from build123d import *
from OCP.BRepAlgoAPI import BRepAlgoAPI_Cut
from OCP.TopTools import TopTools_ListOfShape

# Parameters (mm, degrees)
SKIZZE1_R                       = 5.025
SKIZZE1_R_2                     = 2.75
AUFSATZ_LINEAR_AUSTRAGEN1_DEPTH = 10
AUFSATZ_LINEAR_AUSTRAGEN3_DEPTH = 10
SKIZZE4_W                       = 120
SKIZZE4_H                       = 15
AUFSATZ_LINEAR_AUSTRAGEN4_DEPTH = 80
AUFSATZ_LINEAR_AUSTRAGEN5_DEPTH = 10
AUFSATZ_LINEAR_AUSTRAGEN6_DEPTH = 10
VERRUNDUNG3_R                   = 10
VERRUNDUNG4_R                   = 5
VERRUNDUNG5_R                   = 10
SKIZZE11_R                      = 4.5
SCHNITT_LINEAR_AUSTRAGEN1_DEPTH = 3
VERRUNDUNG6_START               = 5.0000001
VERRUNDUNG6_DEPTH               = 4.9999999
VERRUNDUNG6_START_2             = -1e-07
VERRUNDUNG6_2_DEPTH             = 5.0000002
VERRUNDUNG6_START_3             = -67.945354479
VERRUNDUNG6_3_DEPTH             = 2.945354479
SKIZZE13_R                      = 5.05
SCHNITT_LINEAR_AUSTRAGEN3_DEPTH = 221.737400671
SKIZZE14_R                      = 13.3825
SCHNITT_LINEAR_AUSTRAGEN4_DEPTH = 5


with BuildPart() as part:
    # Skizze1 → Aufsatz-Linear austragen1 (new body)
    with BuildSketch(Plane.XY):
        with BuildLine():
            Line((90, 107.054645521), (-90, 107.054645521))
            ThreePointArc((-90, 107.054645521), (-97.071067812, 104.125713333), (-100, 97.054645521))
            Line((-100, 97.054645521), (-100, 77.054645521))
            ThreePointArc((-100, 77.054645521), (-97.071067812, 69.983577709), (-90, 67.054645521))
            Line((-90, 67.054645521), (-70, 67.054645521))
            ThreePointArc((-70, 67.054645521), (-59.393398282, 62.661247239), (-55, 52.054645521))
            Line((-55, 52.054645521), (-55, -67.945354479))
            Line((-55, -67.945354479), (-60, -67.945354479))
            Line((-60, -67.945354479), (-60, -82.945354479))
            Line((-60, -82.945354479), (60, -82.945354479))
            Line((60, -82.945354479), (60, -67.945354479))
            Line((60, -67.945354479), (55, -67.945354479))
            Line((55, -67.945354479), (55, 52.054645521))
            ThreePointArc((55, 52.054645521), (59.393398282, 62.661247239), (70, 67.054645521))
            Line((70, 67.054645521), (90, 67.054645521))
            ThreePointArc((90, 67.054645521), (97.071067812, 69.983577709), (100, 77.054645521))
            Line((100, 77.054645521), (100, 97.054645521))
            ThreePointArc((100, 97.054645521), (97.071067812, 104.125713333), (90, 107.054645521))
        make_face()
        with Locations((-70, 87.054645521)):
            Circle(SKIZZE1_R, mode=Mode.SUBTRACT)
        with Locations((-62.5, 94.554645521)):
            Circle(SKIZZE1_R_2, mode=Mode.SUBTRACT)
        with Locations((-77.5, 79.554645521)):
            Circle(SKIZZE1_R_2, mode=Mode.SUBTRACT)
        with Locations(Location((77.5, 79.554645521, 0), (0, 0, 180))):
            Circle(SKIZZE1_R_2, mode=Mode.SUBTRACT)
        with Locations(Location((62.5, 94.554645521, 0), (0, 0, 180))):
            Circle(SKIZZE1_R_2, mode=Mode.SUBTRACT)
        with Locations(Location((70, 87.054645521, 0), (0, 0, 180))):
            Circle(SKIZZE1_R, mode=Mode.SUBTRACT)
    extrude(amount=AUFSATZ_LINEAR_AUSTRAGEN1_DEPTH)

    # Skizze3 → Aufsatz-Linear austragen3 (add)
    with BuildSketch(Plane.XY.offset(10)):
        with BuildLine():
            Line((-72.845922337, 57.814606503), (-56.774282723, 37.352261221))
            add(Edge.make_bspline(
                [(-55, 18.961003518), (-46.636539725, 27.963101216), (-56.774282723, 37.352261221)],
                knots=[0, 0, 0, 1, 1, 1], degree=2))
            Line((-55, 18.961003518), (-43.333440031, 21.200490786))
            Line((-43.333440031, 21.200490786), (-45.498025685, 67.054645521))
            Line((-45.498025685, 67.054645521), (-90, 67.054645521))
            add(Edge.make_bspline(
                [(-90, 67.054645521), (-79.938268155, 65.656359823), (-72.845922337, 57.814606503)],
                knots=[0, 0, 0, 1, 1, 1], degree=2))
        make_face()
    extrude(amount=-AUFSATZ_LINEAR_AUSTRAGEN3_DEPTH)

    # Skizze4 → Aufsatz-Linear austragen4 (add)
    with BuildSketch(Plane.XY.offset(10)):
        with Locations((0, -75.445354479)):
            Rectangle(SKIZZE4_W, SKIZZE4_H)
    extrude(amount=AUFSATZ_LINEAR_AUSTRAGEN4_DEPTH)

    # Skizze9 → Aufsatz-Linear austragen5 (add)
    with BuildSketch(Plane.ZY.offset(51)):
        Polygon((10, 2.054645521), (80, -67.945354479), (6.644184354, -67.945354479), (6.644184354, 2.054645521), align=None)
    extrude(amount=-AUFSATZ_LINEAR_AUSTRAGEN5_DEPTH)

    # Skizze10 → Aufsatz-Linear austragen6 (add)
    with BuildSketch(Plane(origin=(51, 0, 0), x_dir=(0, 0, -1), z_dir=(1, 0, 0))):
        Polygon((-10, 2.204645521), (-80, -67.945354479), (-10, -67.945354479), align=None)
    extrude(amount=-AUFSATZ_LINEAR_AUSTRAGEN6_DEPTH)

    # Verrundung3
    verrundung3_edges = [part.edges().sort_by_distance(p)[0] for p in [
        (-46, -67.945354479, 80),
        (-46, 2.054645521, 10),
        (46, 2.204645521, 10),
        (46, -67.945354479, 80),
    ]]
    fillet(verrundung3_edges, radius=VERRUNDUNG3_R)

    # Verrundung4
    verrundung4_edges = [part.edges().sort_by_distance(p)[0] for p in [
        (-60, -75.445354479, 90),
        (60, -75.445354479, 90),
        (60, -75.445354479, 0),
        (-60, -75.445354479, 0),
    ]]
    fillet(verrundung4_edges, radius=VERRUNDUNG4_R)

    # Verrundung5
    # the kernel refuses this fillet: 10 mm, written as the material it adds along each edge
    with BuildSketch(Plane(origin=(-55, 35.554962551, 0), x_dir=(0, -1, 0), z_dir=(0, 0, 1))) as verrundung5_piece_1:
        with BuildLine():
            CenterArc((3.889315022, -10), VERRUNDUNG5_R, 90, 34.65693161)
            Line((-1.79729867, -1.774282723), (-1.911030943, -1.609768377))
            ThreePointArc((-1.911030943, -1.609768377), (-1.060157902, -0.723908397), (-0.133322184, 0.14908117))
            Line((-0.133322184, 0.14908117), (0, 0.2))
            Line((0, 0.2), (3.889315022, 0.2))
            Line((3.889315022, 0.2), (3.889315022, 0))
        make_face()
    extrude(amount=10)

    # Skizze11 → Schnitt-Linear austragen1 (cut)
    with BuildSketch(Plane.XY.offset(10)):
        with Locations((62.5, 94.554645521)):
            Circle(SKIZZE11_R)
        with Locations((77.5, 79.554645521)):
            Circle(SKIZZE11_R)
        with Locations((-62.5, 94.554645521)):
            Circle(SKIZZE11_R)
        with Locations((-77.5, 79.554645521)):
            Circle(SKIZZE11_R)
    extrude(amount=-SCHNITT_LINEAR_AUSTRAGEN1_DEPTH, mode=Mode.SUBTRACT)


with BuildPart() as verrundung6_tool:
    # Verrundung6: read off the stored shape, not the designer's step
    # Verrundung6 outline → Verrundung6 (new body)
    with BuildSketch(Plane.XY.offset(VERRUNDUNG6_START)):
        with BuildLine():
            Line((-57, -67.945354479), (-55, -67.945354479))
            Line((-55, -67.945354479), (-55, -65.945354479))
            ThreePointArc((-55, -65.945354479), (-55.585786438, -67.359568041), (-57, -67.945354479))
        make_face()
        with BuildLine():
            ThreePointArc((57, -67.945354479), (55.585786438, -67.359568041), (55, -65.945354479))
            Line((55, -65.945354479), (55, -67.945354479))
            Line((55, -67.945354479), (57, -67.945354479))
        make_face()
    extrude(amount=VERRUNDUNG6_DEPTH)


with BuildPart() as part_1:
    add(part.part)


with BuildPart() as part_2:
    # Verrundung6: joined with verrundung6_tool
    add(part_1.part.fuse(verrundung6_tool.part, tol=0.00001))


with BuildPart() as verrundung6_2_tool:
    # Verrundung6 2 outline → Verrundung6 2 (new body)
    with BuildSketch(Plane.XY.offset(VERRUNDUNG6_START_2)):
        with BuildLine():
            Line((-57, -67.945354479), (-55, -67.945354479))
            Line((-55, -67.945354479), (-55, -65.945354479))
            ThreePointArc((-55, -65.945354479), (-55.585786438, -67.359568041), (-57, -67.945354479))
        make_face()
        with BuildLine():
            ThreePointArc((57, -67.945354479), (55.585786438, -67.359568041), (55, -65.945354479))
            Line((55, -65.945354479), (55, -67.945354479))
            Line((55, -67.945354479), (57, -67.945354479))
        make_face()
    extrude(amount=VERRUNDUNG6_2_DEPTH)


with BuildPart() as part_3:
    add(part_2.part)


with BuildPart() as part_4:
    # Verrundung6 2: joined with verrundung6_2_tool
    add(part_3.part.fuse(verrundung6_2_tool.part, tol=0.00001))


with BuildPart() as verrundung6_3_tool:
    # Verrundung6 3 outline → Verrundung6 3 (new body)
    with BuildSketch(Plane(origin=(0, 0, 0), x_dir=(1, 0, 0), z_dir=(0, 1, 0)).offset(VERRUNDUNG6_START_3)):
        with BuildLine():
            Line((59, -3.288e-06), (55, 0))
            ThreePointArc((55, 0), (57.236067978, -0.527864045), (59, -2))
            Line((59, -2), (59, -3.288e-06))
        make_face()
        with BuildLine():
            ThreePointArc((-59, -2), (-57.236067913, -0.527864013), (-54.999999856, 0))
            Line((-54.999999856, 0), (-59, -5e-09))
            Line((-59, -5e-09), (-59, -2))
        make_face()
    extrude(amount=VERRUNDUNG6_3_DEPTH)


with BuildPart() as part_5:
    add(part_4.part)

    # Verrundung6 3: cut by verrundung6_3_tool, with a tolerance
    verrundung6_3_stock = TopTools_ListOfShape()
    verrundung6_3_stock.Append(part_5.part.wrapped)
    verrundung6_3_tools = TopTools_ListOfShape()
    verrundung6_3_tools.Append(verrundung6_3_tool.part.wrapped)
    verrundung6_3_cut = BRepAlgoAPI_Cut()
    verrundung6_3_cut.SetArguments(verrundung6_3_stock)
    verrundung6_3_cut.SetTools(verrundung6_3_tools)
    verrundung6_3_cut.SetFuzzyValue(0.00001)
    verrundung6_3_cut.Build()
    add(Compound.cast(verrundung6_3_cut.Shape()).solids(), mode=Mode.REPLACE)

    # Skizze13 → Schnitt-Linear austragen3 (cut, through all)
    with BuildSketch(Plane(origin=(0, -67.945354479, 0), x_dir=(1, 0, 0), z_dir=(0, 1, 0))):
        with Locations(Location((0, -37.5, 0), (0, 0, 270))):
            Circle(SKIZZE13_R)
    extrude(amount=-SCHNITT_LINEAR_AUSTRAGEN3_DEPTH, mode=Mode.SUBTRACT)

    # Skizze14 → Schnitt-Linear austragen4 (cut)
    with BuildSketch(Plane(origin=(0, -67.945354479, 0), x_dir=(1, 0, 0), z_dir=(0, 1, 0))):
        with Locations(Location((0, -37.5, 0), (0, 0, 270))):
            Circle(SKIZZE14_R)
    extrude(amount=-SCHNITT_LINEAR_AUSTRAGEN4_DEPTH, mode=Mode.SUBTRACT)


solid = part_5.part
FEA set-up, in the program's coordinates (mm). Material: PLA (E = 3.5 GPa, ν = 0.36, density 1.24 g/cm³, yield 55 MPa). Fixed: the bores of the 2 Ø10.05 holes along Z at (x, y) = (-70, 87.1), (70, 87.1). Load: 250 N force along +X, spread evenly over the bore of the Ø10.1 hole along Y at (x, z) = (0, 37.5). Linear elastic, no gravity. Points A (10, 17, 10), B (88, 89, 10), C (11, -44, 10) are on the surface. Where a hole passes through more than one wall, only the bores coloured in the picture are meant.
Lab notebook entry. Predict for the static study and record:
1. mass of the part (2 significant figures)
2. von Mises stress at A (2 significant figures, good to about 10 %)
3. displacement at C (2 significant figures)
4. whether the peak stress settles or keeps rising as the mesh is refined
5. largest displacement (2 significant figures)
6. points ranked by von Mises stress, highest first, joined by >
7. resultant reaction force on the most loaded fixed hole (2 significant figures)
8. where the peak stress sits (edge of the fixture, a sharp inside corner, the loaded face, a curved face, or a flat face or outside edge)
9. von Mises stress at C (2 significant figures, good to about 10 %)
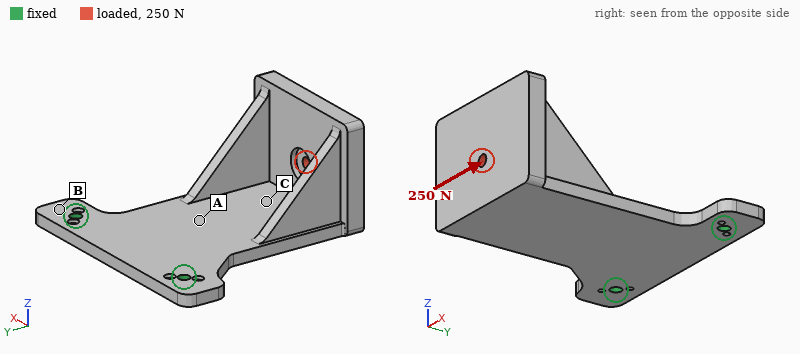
540 g
2.6 MPa
0.23 mm
keeps rising
1.2 mm
A > C > B
330 N
edge of the fixture
1.2 MPa
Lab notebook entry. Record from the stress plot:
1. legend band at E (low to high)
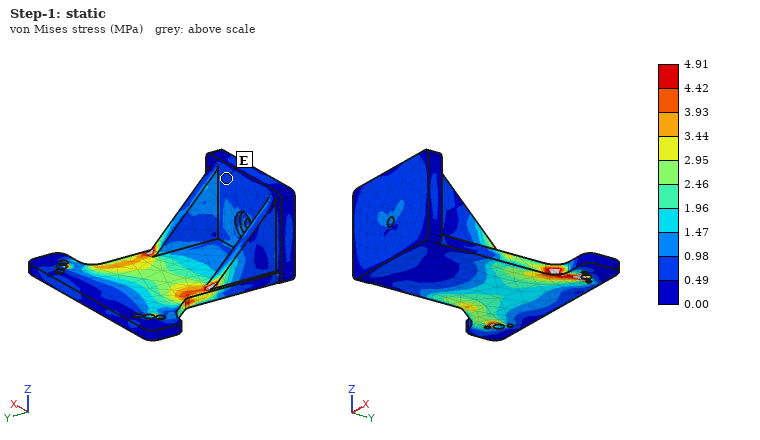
0.49 to 0.98 MPa
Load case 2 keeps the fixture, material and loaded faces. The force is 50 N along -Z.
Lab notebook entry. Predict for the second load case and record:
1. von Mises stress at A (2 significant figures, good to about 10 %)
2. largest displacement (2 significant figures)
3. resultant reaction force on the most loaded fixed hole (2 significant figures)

2.3 MPa
3.3 mm
26 N
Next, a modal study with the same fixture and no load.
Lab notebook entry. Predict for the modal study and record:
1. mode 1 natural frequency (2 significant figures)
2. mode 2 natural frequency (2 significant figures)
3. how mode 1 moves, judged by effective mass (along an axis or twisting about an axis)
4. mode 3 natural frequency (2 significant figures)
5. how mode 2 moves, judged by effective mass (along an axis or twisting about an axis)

40 Hz
140 Hz
along Z
300 Hz
along X
